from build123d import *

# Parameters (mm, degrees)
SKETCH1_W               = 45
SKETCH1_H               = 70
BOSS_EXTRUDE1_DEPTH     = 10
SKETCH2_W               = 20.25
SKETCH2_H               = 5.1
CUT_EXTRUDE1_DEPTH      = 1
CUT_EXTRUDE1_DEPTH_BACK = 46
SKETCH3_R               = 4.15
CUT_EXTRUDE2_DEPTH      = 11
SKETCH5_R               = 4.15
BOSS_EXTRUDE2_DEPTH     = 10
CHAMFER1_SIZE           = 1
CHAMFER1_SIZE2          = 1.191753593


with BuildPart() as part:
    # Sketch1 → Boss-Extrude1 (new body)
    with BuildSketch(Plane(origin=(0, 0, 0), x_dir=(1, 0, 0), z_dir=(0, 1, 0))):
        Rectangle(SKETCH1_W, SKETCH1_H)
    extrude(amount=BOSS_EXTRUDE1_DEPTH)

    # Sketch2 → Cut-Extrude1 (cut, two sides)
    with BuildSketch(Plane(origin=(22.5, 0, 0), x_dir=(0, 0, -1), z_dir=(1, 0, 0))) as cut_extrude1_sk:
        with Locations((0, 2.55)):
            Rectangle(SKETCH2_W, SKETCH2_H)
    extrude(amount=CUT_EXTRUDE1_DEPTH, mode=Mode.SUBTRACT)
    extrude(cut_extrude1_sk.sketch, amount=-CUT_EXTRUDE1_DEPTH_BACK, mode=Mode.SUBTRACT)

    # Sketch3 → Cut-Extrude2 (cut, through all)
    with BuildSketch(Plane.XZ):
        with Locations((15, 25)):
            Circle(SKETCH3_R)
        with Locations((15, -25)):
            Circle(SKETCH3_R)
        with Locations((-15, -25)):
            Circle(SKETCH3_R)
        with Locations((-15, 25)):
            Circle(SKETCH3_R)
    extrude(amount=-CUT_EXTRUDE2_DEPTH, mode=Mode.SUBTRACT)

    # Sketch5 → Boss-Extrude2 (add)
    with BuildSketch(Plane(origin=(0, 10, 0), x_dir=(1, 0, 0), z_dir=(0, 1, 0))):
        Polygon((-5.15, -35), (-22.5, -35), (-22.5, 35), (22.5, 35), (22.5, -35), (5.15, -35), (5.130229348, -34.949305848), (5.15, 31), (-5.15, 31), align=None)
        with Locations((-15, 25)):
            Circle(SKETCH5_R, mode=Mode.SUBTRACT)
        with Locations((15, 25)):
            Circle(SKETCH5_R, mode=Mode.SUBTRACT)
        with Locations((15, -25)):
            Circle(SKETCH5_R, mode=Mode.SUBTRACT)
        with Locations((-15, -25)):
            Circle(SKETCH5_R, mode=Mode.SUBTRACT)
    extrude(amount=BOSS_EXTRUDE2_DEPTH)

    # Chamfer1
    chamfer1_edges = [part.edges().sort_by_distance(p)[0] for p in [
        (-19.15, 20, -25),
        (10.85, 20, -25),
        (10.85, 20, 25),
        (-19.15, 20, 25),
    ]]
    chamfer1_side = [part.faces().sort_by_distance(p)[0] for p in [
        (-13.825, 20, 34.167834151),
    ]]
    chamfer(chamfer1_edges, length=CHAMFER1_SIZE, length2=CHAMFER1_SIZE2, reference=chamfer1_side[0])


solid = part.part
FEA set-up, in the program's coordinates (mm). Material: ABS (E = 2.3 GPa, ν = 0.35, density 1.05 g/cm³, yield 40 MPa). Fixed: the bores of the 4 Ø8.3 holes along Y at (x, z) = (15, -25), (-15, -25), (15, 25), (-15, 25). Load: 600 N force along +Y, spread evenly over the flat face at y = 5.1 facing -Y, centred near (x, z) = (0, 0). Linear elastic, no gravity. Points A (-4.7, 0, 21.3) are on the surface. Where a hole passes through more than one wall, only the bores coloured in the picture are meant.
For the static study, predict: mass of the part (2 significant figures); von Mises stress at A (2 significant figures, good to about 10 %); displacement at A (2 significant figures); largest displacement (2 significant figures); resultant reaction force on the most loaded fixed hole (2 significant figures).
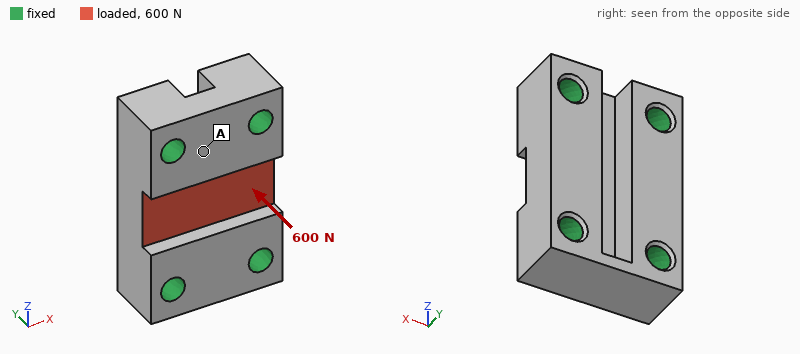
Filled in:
50 g
0.63 MPa
5.5 µm
26 µm
150 N
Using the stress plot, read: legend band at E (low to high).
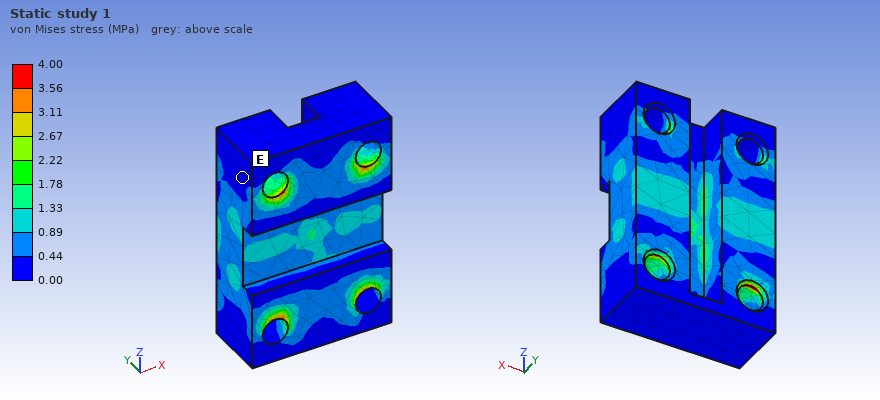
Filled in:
0.00 to 0.44 MPa
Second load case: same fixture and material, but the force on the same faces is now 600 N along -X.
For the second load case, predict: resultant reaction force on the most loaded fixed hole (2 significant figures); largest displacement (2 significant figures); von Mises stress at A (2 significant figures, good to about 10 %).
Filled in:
170 N
25 µm
0.69 MPa
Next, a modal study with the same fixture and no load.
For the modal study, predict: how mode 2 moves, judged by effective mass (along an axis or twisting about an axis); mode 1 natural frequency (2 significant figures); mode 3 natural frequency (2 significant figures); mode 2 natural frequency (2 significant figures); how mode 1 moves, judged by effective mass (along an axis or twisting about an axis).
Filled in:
along X
7600 Hz
8900 Hz
8000 Hz
along Y
